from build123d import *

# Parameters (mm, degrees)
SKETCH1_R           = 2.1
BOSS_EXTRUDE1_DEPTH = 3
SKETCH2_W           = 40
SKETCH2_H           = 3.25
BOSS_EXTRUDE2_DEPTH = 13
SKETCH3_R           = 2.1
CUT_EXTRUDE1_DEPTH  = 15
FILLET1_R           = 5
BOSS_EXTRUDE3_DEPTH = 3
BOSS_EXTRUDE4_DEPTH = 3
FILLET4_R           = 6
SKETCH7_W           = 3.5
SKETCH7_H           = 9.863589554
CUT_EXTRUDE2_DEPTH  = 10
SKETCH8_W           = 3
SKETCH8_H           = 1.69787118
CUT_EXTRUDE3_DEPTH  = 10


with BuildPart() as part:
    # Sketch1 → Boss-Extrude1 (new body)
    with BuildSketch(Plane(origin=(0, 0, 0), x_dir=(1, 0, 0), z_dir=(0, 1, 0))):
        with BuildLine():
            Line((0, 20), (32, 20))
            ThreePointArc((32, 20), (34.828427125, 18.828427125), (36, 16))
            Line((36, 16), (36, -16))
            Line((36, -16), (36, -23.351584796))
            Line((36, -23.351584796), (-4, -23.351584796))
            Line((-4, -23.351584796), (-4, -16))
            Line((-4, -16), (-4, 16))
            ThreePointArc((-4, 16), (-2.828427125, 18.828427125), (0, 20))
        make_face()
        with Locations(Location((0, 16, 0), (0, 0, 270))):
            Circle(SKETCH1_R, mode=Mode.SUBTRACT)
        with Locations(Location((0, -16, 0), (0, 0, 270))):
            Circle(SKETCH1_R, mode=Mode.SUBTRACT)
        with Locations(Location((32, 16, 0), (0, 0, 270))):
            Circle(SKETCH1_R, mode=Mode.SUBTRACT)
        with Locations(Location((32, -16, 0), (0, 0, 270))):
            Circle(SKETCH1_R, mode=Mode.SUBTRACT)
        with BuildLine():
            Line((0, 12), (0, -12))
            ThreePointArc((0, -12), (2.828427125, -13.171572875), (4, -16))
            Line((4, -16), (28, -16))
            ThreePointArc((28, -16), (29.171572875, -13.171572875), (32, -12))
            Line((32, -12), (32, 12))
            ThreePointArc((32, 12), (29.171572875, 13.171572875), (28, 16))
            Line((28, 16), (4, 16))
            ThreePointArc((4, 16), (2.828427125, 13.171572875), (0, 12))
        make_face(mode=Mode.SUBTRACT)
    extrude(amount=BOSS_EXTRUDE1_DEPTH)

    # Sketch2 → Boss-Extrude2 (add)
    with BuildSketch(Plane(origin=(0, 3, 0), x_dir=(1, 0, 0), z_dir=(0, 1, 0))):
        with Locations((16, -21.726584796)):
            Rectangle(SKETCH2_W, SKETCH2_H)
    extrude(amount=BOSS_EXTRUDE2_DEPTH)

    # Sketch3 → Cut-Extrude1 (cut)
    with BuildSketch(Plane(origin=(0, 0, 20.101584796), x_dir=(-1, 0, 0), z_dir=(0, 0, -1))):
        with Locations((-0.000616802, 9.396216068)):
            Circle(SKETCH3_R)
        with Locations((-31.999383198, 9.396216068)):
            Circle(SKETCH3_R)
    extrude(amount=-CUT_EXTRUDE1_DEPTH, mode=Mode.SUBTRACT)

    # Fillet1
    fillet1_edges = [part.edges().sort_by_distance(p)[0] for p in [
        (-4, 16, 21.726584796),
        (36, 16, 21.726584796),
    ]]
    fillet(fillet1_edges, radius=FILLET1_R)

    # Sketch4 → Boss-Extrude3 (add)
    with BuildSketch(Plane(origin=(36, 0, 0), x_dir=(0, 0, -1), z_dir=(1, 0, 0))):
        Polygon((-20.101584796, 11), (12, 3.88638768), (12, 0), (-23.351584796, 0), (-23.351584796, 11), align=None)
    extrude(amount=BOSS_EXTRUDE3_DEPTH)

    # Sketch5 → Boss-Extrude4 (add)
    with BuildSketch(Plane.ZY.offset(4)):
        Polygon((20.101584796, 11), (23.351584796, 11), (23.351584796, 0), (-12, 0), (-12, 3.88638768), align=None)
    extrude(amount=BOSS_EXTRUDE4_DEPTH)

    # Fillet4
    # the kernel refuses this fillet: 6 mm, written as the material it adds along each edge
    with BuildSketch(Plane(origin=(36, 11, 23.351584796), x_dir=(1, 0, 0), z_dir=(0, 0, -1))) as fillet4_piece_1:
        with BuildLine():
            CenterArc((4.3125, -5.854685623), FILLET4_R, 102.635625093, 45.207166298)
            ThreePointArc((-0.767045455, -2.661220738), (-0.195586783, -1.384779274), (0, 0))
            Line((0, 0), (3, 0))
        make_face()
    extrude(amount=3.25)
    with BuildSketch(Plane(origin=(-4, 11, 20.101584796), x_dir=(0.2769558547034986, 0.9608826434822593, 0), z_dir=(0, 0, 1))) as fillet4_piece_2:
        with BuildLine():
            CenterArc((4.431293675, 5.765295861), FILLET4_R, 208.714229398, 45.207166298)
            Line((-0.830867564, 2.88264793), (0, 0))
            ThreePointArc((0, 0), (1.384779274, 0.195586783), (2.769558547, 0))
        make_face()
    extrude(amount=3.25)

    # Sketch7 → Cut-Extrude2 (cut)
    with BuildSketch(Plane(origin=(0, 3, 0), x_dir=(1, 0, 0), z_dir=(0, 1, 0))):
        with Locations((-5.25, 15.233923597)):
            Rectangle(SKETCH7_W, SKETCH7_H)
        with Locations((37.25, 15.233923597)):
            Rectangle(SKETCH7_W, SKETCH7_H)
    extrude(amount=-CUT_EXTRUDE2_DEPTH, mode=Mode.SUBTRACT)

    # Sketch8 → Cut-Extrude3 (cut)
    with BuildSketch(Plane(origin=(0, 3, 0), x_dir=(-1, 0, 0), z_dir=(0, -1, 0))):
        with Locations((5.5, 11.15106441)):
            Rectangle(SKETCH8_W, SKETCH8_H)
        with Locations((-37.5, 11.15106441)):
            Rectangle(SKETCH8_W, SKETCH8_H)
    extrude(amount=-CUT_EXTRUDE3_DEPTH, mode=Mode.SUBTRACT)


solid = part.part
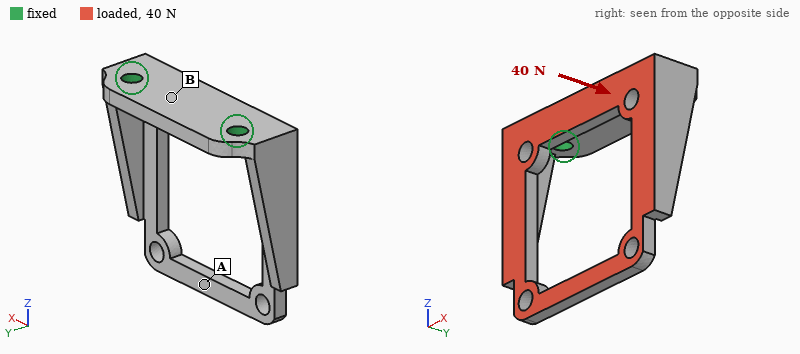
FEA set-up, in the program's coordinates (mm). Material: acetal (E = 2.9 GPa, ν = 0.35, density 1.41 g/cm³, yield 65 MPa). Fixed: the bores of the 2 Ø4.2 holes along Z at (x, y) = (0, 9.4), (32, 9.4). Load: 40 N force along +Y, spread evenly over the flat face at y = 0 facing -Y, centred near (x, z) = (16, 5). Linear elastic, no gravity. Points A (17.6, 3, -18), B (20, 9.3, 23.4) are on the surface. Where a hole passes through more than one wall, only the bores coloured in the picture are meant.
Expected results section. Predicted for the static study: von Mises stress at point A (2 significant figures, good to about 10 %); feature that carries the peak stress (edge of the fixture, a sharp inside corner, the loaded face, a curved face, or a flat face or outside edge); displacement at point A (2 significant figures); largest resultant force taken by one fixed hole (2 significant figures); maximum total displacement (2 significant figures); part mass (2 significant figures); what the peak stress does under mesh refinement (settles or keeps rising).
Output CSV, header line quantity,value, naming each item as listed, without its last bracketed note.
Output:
quantity,value
von Mises stress at point A,3.7 MPa
feature that carries the peak stress,edge of the fixture
displacement at point A,0.69 mm
largest resultant force taken by one fixed hole,20 N
maximum total displacement,0.75 mm
part mass,7.4 g
what the peak stress does under mesh refinement,keeps rising
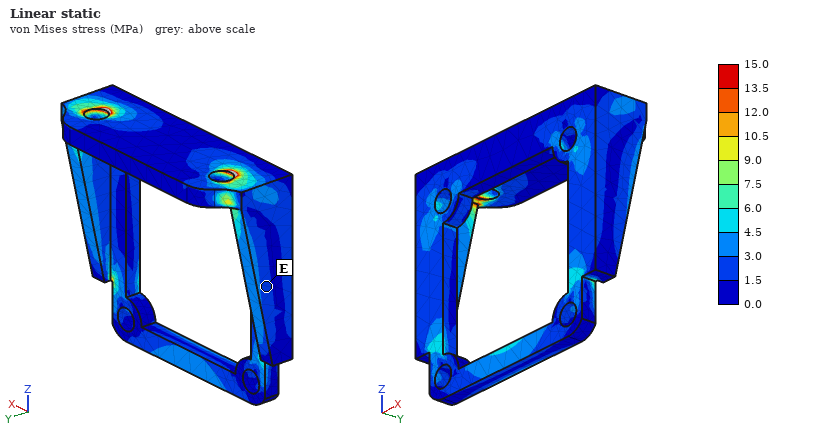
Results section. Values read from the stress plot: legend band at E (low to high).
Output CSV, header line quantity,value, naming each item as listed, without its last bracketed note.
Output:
quantity,value
legend band at E,1.5 to 3.0 MPa
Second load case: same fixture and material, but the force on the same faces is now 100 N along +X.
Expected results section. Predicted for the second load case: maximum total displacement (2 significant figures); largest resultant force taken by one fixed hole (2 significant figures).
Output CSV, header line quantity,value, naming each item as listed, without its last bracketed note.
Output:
quantity,value
maximum total displacement,0.71 mm
largest resultant force taken by one fixed hole,68 N
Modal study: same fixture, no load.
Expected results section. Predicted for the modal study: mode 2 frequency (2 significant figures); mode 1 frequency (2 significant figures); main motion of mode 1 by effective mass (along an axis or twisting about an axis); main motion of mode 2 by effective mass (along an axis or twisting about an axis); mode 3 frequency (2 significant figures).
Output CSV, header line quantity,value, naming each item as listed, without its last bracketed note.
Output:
quantity,value
mode 2 frequency,910 Hz
mode 1 frequency,720 Hz
main motion of mode 1 by effective mass,along Y
main motion of mode 2 by effective mass,along X
mode 3 frequency,1400 Hz
